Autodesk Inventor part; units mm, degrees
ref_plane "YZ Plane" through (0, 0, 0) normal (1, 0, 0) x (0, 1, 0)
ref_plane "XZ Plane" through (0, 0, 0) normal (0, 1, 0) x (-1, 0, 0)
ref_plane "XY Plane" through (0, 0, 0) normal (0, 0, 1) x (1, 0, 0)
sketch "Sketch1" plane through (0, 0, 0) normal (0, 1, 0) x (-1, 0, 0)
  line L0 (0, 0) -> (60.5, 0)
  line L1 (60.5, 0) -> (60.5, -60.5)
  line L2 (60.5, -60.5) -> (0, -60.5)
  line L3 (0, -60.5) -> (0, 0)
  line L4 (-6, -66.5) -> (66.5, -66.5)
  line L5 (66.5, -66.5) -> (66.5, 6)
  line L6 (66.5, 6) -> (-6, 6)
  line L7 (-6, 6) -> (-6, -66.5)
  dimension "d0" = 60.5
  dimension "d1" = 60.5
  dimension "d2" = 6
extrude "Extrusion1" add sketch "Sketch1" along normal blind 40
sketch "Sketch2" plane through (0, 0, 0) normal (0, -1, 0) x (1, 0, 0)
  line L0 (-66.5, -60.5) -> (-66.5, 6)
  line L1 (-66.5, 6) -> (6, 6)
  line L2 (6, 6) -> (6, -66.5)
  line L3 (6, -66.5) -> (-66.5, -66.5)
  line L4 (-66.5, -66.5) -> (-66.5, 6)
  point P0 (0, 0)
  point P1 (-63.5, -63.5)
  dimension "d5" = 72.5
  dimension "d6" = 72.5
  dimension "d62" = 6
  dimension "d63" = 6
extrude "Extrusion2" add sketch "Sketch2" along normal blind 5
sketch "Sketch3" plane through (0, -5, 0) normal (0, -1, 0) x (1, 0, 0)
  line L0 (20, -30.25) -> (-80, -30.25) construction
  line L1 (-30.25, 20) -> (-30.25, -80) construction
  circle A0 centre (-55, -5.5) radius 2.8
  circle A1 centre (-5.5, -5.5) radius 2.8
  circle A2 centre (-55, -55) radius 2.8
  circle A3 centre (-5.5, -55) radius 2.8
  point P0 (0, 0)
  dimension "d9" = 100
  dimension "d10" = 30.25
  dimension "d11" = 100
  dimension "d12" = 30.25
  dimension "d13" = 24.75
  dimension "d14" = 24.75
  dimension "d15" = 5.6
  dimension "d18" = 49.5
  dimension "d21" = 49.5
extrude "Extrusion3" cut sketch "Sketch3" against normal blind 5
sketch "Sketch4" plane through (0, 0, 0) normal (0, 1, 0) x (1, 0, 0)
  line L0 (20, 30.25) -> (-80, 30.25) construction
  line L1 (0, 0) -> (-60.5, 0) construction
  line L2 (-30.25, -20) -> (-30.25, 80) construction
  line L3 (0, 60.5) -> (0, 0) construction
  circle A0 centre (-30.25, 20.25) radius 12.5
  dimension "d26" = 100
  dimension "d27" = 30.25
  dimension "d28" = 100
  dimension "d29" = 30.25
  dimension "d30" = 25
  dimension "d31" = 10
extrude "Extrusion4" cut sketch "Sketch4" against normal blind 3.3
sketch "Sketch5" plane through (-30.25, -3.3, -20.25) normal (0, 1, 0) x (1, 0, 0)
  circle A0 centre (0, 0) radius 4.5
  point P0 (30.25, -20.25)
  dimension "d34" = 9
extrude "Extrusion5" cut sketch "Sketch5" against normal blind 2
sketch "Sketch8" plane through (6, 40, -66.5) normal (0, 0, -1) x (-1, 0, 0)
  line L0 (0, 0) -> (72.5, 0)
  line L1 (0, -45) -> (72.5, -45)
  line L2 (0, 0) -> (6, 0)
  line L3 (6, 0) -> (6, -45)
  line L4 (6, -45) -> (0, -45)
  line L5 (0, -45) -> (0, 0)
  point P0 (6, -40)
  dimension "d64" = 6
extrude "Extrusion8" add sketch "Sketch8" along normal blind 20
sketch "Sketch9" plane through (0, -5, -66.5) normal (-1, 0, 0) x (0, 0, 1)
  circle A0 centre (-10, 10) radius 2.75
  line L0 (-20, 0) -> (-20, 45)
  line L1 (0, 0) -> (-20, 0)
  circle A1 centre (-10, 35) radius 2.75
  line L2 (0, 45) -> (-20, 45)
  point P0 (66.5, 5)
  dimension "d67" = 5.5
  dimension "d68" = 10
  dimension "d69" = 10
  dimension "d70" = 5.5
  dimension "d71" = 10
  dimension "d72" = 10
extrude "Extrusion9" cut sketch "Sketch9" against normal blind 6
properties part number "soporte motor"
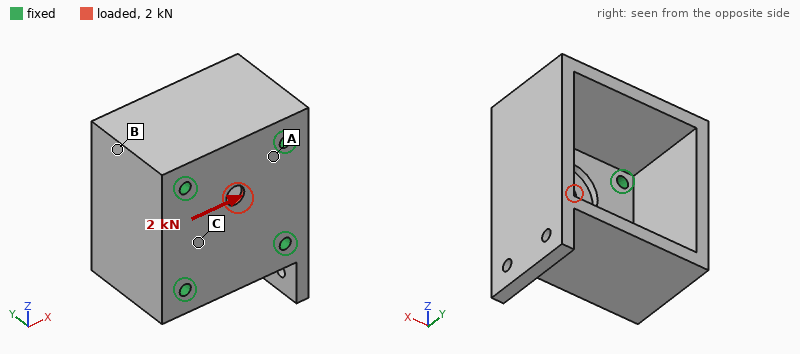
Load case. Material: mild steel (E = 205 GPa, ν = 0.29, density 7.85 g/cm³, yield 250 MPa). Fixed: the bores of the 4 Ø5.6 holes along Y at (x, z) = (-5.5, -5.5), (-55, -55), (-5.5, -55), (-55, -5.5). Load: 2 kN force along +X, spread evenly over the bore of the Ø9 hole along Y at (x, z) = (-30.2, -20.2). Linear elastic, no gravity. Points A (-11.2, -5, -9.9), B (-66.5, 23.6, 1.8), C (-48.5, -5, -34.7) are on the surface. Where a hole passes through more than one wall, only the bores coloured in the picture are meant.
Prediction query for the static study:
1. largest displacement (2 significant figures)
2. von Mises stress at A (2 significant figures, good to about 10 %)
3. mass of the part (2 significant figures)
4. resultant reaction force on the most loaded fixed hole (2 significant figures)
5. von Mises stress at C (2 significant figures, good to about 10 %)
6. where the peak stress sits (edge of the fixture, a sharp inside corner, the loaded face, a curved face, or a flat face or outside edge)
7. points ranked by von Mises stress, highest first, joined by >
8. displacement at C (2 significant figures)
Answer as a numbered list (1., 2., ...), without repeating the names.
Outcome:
1. 2.8 µm
2. 13 MPa
3. 730 g
4. 680 N
5. 6.1 MPa
6. the loaded face
7. A > C > B
8. 0.66 µm
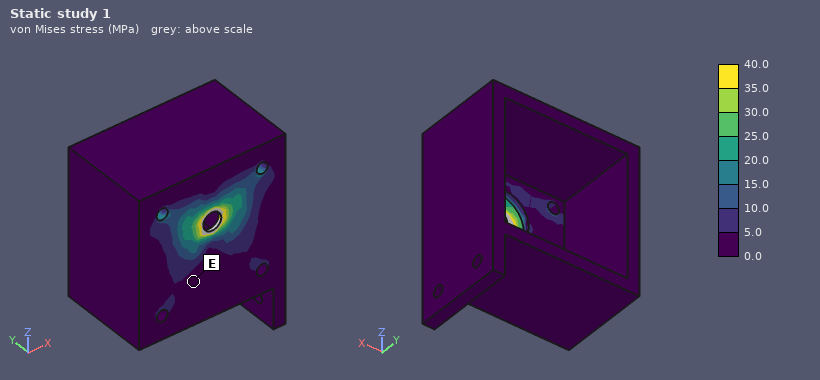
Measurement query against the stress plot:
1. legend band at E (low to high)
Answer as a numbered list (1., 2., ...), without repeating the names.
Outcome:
1. 0.0 to 5.0 MPa
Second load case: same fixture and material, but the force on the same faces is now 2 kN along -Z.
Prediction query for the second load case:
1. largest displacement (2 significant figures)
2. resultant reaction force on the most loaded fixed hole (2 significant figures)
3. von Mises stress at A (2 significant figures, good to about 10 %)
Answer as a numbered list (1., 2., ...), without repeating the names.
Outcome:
1. 3.2 µm
2. 600 N
3. 8.7 MPa
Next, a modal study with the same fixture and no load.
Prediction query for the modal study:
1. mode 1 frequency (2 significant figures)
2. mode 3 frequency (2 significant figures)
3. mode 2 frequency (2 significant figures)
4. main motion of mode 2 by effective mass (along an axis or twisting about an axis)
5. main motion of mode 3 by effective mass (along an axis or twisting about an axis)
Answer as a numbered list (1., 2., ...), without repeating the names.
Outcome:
1. 4800 Hz
2. 5500 Hz
3. 5200 Hz
4. along Z
5. along X
